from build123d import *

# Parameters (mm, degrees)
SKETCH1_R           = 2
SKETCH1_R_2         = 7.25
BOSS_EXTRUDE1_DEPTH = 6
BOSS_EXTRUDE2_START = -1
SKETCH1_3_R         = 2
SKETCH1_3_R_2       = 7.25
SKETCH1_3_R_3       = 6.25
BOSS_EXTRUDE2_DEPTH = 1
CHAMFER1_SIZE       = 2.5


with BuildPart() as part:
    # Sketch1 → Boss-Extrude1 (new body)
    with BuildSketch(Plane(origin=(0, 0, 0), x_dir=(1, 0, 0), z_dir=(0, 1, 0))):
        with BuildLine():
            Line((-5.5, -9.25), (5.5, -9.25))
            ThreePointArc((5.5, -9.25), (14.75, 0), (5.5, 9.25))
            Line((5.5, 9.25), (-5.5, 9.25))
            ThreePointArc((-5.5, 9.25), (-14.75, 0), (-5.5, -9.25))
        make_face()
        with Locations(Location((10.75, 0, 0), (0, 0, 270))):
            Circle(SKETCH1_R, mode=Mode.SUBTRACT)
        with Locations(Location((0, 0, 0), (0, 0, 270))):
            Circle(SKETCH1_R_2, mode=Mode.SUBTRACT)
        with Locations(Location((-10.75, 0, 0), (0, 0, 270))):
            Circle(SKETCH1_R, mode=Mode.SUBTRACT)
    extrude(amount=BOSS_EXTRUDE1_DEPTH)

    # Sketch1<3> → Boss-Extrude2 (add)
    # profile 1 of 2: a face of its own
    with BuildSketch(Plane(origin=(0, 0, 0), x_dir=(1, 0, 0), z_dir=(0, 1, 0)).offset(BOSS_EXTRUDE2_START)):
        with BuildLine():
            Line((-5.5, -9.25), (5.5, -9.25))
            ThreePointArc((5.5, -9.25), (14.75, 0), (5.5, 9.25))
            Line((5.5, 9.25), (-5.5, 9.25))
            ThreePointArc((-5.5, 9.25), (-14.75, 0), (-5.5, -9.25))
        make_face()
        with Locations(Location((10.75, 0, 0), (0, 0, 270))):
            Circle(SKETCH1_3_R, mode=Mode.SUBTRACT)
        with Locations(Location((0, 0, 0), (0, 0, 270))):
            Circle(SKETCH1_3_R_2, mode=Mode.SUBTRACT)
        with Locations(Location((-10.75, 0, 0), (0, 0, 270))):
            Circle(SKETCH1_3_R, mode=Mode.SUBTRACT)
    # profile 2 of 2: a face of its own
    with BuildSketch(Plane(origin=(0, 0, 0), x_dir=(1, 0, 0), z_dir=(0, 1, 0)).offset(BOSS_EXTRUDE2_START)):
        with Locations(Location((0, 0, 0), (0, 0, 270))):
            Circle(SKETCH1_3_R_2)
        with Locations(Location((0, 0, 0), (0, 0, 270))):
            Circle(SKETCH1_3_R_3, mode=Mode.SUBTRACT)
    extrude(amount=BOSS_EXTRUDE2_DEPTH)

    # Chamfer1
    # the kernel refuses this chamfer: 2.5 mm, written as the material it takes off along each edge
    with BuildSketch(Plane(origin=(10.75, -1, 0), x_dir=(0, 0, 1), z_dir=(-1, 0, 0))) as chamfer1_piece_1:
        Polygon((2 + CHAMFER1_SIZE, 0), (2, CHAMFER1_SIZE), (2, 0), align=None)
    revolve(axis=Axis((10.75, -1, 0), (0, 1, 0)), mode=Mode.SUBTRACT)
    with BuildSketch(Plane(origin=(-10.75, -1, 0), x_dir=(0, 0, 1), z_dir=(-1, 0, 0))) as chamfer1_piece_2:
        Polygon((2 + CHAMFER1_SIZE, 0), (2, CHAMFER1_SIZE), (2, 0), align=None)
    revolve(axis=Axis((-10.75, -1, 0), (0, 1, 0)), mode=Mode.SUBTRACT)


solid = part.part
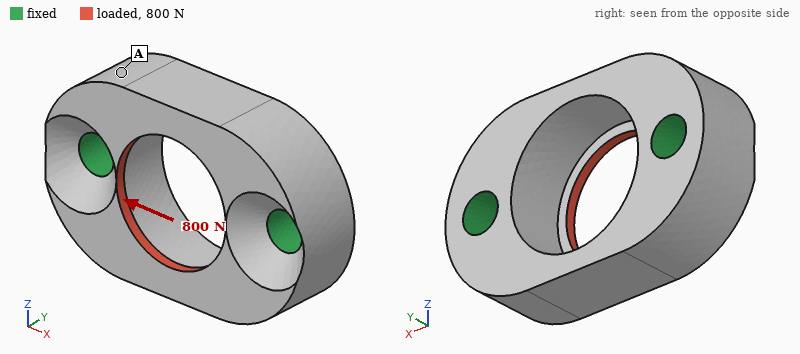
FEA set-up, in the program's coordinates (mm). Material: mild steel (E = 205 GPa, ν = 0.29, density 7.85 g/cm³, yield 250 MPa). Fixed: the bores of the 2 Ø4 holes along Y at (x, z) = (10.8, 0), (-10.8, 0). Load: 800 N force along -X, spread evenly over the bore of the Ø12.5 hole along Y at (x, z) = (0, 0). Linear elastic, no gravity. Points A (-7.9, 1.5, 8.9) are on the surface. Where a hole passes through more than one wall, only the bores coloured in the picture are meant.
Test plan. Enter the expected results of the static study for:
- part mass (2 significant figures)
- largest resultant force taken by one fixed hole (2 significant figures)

15 g
410 N
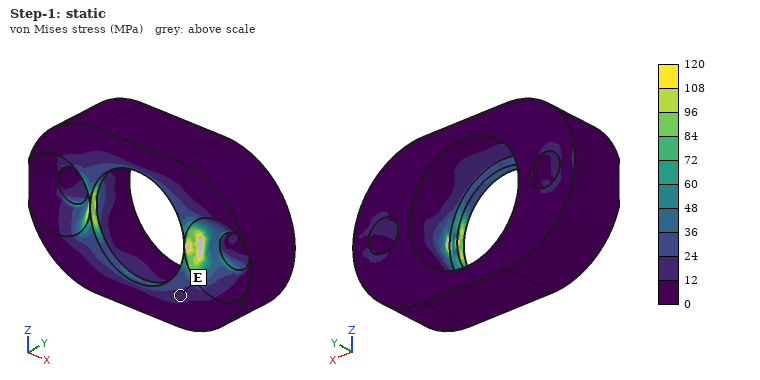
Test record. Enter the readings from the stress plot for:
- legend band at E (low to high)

12 to 24 MPa
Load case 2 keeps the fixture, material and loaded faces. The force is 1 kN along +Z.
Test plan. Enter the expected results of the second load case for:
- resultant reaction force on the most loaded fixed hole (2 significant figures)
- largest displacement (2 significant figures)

500 N
4.2 µm
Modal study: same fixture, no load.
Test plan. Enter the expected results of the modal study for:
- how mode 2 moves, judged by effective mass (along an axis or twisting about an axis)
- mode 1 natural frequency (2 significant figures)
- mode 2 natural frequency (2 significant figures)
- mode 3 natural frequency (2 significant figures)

along Y
31 kHz
34 kHz
47 kHz
